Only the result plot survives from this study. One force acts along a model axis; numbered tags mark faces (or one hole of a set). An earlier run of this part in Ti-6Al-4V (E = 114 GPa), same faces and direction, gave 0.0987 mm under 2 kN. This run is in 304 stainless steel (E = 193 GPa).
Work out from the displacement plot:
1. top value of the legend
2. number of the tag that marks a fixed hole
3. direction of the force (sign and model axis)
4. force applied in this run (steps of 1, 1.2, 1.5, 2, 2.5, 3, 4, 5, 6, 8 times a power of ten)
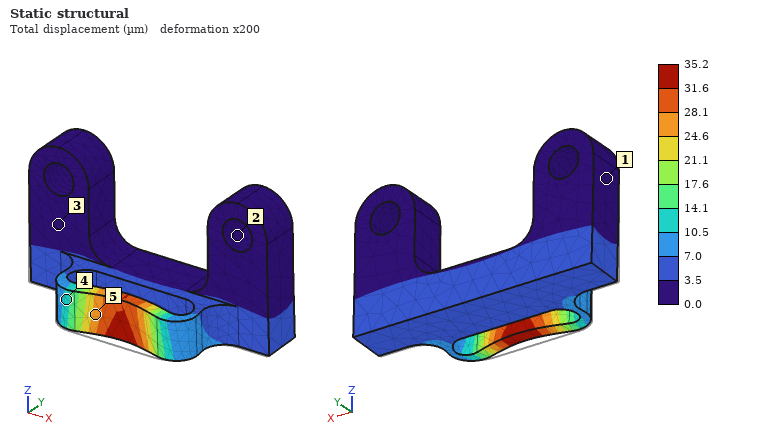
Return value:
35.2 µm
2
+Y
1.2 kN
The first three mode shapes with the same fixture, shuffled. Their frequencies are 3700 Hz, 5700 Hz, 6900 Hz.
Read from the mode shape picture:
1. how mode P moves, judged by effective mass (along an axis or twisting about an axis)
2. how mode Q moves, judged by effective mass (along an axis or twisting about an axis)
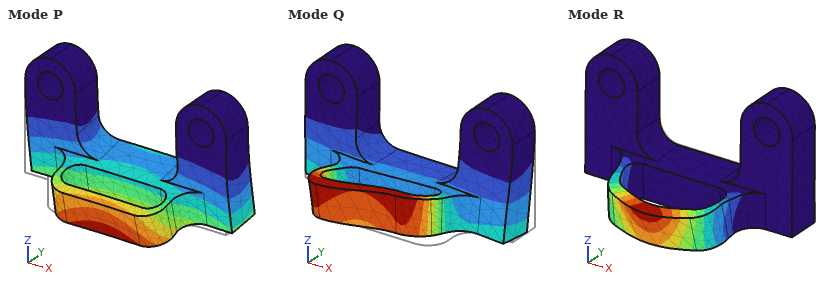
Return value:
along Y
along X
